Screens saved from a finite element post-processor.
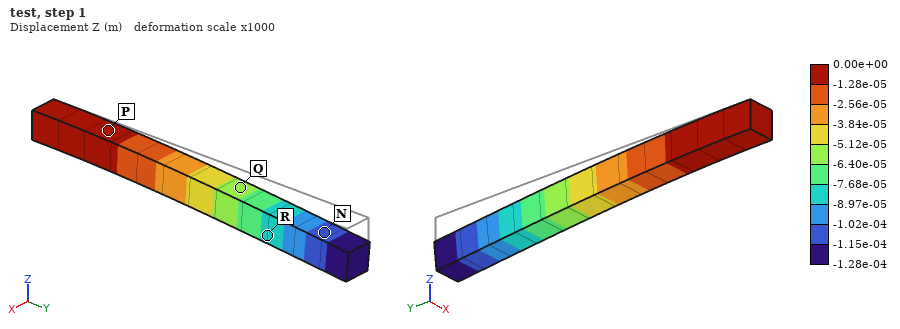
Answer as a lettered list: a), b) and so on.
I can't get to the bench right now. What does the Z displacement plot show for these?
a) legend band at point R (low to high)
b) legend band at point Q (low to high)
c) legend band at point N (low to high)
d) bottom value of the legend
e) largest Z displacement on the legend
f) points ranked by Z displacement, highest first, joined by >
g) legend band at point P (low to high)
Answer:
a) -8.97e-05 to -7.68e-05 m
b) -6.40e-05 to -5.12e-05 m
c) -1.15e-04 to -1.02e-04 m
d) -1.28e-04 m
e) 0.00e+00 m
f) P > Q > R > N
g) -1.28e-05 to 0.00e+00 m
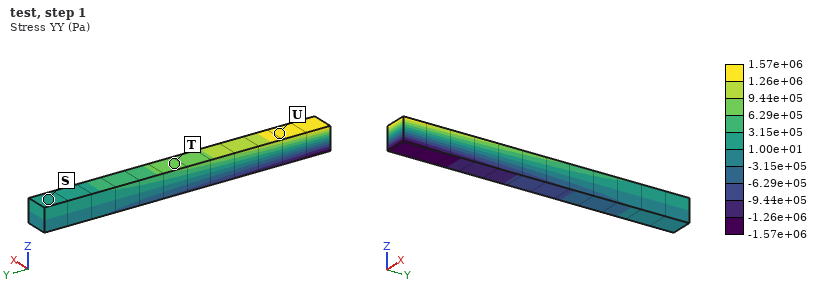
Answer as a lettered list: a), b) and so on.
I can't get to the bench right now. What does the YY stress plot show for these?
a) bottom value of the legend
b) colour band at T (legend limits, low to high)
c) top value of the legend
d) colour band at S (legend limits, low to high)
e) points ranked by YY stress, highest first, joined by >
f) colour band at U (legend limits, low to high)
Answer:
a) -1.57e+06 Pa
b) 6.29e+05 to 9.44e+05 Pa
c) 1.57e+06 Pa
d) 1.00e+01 to 3.15e+05 Pa
e) U > T > S
f) 1.26e+06 to 1.57e+06 Pa
